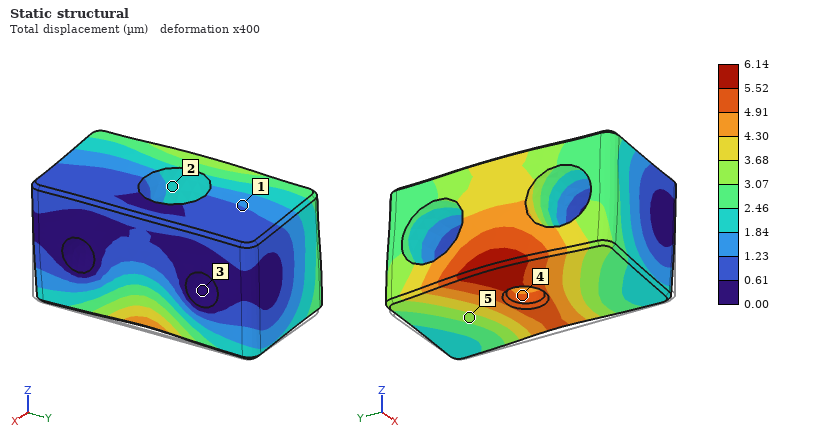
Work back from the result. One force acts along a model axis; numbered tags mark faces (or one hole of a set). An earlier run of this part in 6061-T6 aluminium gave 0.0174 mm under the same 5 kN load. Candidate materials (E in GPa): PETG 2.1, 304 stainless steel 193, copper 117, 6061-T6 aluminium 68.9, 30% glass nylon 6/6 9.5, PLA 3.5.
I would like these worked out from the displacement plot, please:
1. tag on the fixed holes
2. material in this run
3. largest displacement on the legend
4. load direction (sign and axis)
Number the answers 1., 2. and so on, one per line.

1. 3
2. 304 stainless steel
3. 6.14 µm
4. -X
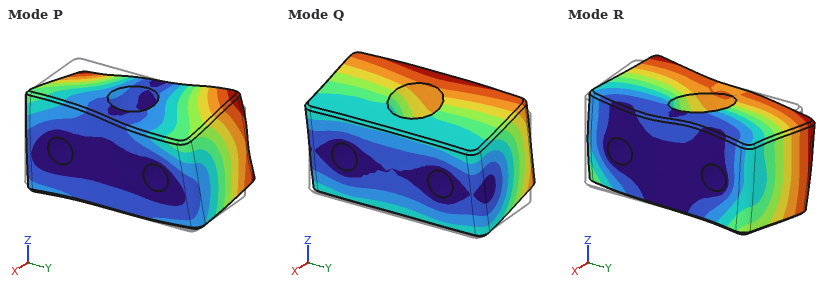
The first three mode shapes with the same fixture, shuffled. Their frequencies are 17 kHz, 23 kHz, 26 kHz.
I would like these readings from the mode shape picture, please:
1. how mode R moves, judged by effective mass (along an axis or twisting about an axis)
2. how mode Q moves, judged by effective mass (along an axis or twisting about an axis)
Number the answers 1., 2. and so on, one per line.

1. along Y
2. along Z
